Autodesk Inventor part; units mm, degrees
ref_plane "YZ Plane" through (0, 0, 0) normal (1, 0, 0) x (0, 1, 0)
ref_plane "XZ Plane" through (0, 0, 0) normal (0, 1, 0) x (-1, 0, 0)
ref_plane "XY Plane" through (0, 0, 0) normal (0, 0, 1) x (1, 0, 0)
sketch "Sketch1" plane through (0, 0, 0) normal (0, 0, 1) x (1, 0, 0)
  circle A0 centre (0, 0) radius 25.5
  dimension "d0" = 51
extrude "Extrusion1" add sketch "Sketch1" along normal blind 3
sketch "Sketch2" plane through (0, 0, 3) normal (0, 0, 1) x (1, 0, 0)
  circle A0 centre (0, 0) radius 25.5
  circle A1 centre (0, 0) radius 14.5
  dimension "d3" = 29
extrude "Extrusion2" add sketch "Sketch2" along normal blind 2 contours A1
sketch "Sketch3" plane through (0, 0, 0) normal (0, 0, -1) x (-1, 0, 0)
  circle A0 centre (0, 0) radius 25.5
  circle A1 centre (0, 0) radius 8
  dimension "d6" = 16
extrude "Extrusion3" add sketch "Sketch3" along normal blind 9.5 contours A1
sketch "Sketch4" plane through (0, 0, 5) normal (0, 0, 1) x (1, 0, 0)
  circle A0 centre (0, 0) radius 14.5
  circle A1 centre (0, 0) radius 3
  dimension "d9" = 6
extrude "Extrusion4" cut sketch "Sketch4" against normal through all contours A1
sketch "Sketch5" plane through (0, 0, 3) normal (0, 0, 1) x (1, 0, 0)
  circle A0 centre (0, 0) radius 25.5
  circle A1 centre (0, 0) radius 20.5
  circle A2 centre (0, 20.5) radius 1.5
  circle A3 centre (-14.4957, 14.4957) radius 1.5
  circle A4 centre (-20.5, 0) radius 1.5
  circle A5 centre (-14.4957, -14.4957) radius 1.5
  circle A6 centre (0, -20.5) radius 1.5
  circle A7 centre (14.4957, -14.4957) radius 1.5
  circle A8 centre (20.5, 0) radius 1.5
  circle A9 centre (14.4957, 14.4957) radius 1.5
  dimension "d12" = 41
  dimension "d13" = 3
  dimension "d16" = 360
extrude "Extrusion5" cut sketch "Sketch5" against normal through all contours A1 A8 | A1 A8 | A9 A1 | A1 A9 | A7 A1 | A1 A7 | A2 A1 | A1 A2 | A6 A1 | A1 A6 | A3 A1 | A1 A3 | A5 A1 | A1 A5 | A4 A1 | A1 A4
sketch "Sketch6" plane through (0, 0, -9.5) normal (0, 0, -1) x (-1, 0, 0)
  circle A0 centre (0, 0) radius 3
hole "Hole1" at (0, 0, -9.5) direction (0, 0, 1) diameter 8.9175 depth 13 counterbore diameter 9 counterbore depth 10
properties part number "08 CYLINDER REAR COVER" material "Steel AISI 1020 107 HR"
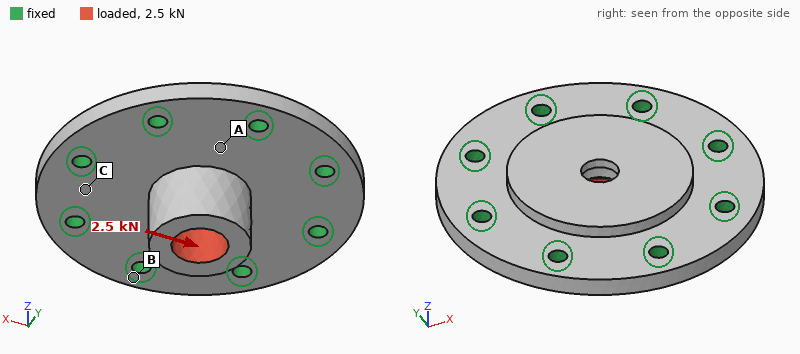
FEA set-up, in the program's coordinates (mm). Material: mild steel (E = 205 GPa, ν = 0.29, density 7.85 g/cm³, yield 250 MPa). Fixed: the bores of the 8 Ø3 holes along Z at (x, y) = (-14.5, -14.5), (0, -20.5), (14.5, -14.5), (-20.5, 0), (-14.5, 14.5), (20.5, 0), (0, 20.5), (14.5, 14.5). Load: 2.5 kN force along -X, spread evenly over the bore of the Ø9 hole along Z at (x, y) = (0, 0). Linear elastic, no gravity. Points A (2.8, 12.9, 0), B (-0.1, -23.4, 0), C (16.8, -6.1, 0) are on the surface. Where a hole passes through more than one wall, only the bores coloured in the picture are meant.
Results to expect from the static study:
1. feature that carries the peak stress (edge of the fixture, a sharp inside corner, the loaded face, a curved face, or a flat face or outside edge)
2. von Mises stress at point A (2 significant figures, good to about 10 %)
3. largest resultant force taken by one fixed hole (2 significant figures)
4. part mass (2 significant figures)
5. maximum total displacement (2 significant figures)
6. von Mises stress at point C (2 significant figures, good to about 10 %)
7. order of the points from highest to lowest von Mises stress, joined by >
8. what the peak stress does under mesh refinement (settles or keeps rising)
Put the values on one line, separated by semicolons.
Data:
edge of the fixture; 24 MPa; 510 N; 65 g; 9.2 µm; 13 MPa; A > C > B; keeps rising
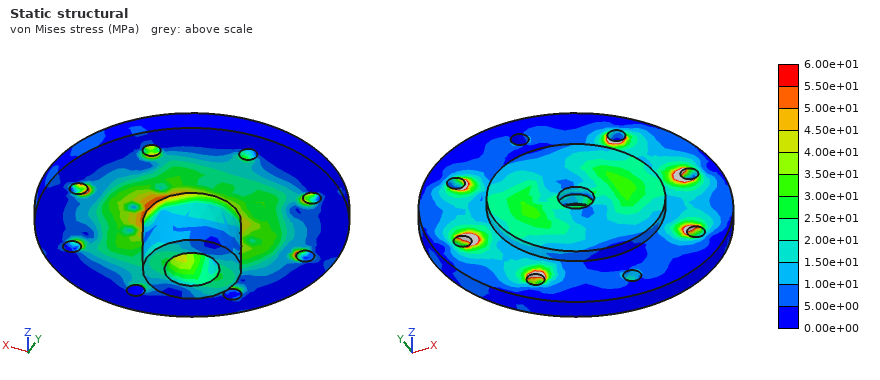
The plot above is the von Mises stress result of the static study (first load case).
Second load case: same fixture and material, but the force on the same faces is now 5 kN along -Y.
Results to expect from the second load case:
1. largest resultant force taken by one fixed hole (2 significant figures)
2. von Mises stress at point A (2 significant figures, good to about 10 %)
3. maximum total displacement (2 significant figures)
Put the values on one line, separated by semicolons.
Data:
1.0 kN; 64 MPa; 19 µm
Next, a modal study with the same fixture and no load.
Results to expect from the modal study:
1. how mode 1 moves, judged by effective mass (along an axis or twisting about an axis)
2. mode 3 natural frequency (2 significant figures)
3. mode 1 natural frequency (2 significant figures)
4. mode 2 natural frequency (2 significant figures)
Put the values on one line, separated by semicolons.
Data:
along Z; 24 kHz; 17 kHz; 24 kHz
